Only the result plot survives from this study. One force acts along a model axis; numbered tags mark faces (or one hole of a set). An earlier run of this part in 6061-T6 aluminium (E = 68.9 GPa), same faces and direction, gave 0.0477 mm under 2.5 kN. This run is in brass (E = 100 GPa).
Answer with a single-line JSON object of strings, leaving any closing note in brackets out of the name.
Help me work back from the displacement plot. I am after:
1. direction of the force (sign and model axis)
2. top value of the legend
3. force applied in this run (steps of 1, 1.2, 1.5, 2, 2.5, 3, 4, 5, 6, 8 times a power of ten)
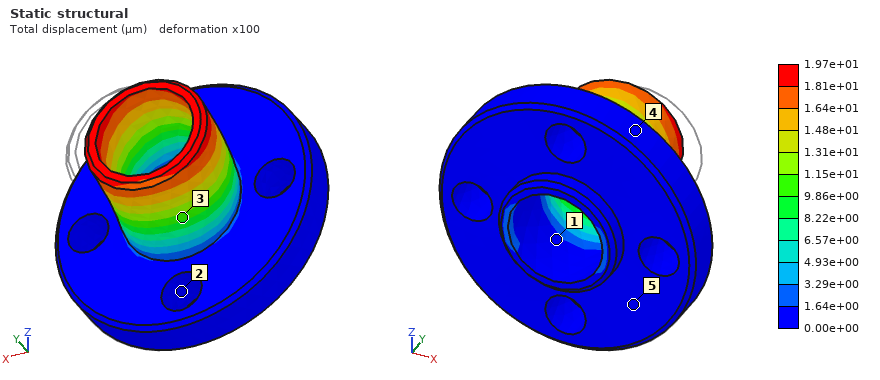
{"direction of the force": "-X", "top value of the legend": "1.97e+01 µm", "force applied in this run": "1.5 kN"}
